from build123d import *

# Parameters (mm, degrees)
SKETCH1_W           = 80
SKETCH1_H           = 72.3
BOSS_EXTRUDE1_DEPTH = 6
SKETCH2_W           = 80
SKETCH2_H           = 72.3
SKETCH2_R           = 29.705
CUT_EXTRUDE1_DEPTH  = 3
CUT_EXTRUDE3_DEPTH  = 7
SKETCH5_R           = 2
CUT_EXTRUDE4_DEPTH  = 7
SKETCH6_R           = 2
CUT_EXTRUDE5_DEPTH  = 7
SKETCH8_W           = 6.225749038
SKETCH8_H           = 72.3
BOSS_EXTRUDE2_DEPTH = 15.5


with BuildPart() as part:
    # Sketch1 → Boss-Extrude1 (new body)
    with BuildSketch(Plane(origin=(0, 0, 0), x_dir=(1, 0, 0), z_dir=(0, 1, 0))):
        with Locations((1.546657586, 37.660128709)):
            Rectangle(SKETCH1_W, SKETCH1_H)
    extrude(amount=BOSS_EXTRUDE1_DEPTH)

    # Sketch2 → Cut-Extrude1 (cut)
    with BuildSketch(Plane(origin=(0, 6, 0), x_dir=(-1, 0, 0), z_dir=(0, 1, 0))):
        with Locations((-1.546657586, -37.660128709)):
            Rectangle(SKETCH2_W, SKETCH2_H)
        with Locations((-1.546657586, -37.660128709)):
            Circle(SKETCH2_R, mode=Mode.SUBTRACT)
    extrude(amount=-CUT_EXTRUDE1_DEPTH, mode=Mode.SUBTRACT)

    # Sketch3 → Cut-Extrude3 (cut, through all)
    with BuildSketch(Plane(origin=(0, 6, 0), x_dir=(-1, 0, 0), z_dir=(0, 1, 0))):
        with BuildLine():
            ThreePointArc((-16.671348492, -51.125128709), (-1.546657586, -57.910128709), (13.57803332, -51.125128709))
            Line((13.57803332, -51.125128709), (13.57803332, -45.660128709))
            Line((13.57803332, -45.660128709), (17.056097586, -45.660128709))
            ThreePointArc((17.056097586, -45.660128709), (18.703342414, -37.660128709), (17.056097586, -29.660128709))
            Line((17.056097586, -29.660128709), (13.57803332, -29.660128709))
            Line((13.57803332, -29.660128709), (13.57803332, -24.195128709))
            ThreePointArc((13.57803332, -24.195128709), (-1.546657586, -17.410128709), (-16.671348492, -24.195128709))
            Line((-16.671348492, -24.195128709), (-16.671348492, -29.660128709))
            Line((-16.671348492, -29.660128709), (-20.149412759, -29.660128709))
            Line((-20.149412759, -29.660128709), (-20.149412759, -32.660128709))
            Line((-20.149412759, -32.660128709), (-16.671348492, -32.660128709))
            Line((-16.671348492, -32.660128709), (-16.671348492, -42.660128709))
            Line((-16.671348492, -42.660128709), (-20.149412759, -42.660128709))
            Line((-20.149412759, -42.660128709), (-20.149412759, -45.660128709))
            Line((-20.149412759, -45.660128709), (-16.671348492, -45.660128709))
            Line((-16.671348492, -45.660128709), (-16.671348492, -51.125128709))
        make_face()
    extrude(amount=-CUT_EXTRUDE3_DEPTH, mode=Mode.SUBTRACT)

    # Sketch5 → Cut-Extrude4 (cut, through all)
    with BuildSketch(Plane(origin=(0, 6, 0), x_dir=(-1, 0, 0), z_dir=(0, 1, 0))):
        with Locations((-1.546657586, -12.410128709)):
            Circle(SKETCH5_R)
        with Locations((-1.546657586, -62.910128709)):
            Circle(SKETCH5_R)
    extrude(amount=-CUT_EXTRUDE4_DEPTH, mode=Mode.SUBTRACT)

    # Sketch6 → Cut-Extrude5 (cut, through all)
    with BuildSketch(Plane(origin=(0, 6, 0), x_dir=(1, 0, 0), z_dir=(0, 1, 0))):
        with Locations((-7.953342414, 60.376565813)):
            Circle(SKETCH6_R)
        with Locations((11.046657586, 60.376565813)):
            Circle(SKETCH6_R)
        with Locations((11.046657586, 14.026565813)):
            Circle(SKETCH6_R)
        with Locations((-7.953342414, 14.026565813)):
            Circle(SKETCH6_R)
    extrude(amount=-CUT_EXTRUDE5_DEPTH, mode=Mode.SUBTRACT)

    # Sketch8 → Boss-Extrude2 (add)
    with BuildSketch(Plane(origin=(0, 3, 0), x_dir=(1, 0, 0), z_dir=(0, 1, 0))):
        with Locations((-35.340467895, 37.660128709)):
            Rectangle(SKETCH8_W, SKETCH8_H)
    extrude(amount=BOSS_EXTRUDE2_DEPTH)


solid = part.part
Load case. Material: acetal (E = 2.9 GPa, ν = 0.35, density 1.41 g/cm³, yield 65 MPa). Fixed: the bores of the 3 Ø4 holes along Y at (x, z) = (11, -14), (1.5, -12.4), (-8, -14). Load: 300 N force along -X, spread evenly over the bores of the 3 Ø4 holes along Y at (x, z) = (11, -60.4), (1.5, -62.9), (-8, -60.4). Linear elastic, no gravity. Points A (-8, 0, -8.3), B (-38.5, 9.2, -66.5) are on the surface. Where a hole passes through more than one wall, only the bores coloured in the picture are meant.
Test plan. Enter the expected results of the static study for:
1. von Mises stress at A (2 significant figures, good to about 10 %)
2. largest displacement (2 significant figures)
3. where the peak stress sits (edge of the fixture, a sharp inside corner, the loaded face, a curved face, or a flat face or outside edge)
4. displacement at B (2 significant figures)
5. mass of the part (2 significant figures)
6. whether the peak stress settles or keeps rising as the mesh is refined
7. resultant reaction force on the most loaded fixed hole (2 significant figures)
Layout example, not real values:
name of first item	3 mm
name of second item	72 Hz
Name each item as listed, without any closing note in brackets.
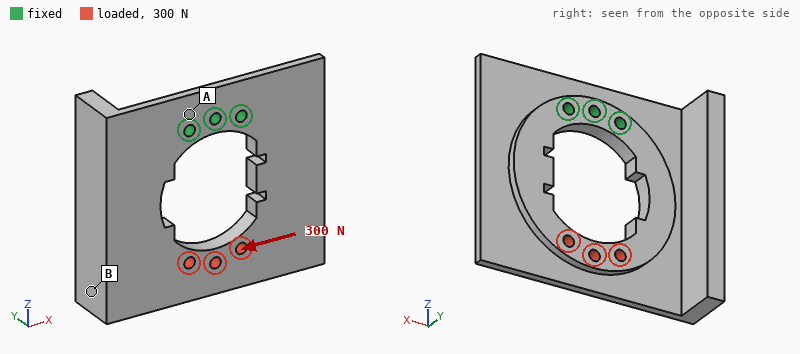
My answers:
von Mises stress at A	13 MPa
largest displacement	1.2 mm
where the peak stress sits	edge of the fixture
displacement at B	1.1 mm
mass of the part	35 g
whether the peak stress settles or keeps rising as the mesh is refined	keeps rising
resultant reaction force on the most loaded fixed hole	530 N
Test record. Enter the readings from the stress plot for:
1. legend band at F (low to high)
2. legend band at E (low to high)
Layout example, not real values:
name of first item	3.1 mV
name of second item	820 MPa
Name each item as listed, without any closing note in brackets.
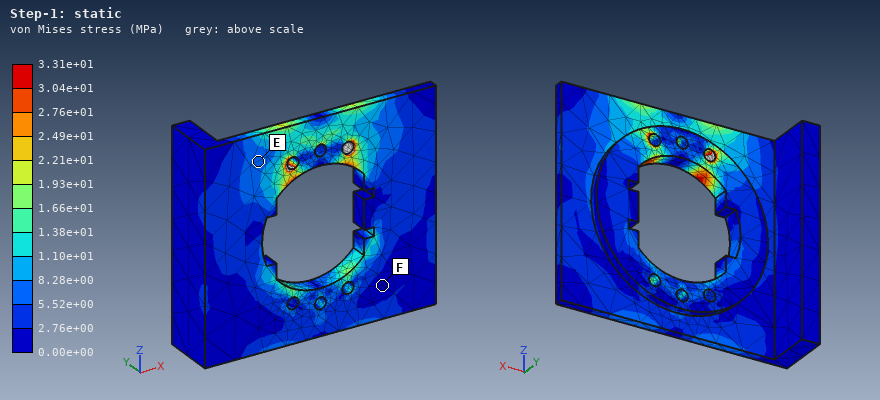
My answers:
legend band at F	0.00e+00 to 2.76e+00 MPa
legend band at E	5.52e+00 to 8.28e+00 MPa
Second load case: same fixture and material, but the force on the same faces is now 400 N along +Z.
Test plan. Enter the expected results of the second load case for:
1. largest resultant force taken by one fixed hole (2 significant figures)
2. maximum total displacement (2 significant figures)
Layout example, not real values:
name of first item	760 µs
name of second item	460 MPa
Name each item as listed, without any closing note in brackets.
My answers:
largest resultant force taken by one fixed hole	250 N
maximum total displacement	0.24 mm
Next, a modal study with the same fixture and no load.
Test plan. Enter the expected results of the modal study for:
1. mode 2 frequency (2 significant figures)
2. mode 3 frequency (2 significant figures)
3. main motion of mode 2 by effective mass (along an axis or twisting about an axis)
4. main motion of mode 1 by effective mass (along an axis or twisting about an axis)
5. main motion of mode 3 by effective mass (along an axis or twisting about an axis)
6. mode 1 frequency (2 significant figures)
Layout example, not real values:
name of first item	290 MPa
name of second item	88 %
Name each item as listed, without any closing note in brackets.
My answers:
mode 2 frequency	340 Hz
mode 3 frequency	560 Hz
main motion of mode 2 by effective mass	twisting about Z
main motion of mode 1 by effective mass	along Y
main motion of mode 3 by effective mass	along X
mode 1 frequency	220 Hz
